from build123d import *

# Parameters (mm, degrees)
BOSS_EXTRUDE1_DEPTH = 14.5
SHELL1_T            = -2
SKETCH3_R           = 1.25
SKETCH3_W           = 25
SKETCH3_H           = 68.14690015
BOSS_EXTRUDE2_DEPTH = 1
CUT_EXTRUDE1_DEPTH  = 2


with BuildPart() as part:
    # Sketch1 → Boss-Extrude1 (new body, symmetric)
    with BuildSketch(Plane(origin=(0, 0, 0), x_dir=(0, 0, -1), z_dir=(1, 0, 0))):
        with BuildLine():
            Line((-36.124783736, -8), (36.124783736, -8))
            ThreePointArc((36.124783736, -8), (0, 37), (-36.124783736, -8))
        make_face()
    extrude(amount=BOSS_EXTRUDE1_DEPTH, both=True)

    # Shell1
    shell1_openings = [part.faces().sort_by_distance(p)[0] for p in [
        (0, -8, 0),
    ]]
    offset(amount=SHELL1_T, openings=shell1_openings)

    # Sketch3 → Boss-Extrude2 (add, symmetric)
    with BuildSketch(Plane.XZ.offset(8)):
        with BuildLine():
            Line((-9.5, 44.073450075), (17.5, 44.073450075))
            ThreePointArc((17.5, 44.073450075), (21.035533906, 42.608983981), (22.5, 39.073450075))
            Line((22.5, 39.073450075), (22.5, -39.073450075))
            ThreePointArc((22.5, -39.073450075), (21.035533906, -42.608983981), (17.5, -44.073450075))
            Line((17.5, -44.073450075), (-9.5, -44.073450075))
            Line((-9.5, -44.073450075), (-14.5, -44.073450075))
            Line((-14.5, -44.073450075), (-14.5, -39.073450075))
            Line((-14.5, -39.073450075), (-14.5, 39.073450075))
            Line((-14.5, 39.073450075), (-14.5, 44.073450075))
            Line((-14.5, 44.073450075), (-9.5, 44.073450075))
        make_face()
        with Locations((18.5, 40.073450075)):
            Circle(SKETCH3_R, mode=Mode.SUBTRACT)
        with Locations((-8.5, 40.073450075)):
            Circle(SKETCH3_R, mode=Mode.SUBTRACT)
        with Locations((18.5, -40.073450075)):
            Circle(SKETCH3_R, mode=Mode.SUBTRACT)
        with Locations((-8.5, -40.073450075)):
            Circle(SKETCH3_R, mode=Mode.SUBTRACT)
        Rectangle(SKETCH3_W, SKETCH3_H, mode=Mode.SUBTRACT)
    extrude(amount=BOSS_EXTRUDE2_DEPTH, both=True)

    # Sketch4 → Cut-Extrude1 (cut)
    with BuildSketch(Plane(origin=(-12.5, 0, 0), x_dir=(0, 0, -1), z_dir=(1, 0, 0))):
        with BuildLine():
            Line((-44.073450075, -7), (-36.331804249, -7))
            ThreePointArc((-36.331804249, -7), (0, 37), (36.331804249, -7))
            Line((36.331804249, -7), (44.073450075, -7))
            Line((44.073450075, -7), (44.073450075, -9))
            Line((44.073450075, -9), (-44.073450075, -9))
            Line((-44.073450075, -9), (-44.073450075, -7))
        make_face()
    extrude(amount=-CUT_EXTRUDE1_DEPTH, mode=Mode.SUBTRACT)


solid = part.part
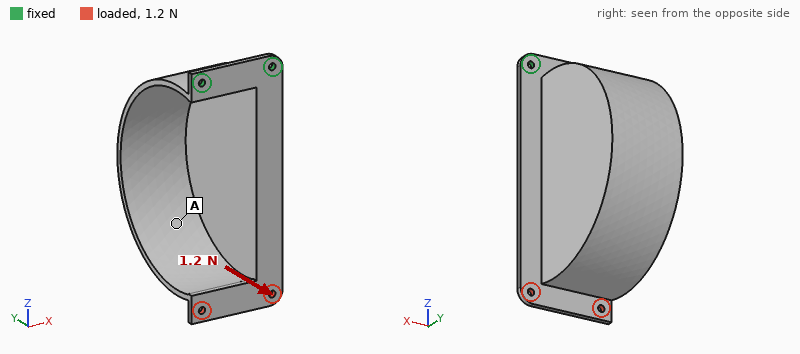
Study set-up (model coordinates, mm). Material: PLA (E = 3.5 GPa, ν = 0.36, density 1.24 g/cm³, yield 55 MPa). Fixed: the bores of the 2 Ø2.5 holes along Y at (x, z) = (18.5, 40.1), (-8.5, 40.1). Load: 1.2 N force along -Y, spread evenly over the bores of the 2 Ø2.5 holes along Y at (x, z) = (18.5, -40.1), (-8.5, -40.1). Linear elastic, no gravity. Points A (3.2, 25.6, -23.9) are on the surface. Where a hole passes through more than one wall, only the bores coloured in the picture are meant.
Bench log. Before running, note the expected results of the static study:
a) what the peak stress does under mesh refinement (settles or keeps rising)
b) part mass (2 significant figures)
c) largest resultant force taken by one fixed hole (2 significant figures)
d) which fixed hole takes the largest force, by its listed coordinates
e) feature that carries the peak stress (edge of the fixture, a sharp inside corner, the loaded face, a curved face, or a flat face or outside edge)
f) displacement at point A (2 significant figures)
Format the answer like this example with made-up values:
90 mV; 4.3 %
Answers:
keeps rising; 18 g; 0.76 N; (18.5, 40.1); edge of the fixture; 0.85 mm
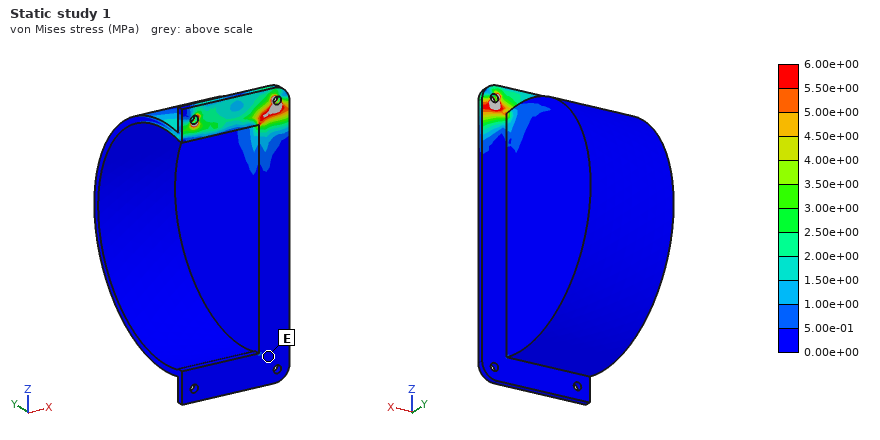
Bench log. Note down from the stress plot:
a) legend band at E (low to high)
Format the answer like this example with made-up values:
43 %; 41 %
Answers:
0.00e+00 to 5.00e-01 MPa
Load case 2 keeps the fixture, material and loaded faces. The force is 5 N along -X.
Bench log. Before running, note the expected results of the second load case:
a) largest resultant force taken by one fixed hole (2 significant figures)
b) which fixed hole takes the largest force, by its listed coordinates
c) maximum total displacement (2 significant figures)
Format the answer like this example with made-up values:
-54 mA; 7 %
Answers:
18 N; (-8.5, 40.1); 1.1 mm
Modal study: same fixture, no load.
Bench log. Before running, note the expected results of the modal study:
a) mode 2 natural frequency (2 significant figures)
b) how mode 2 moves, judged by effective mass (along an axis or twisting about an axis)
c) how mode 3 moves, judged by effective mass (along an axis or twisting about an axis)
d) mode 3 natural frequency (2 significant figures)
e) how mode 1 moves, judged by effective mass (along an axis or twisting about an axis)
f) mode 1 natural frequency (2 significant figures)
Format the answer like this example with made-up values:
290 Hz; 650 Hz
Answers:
160 Hz; along X; twisting about Z; 380 Hz; along Y; 65 Hz
